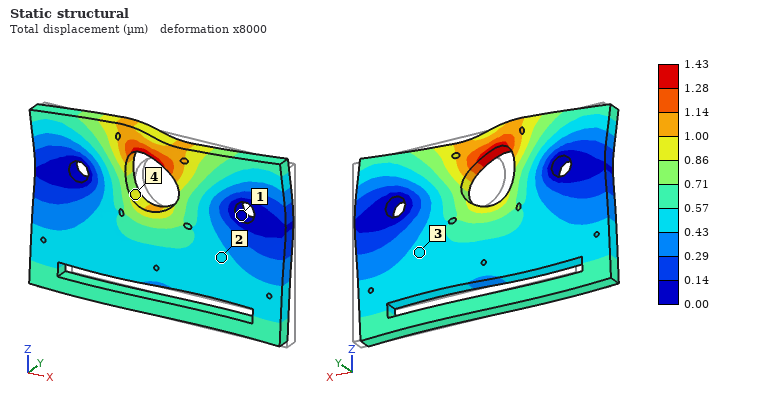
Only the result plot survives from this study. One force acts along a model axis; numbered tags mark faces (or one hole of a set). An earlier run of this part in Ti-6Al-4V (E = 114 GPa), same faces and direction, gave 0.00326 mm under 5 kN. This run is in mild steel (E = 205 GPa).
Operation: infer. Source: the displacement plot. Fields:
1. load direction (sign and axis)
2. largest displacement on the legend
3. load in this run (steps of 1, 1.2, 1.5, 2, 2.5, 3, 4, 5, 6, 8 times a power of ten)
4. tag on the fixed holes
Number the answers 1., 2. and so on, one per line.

1. -X
2. 1.43 µm
3. 4 kN
4. 1
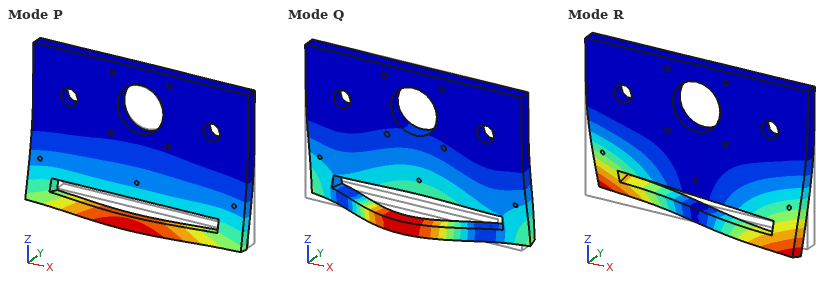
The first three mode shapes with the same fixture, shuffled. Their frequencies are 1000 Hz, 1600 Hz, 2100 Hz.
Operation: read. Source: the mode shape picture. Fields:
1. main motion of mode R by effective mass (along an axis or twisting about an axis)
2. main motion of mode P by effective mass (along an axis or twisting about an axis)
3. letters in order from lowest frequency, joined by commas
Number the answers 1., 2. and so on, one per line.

1. twisting about Z
2. along Y
3. P, R, Q
